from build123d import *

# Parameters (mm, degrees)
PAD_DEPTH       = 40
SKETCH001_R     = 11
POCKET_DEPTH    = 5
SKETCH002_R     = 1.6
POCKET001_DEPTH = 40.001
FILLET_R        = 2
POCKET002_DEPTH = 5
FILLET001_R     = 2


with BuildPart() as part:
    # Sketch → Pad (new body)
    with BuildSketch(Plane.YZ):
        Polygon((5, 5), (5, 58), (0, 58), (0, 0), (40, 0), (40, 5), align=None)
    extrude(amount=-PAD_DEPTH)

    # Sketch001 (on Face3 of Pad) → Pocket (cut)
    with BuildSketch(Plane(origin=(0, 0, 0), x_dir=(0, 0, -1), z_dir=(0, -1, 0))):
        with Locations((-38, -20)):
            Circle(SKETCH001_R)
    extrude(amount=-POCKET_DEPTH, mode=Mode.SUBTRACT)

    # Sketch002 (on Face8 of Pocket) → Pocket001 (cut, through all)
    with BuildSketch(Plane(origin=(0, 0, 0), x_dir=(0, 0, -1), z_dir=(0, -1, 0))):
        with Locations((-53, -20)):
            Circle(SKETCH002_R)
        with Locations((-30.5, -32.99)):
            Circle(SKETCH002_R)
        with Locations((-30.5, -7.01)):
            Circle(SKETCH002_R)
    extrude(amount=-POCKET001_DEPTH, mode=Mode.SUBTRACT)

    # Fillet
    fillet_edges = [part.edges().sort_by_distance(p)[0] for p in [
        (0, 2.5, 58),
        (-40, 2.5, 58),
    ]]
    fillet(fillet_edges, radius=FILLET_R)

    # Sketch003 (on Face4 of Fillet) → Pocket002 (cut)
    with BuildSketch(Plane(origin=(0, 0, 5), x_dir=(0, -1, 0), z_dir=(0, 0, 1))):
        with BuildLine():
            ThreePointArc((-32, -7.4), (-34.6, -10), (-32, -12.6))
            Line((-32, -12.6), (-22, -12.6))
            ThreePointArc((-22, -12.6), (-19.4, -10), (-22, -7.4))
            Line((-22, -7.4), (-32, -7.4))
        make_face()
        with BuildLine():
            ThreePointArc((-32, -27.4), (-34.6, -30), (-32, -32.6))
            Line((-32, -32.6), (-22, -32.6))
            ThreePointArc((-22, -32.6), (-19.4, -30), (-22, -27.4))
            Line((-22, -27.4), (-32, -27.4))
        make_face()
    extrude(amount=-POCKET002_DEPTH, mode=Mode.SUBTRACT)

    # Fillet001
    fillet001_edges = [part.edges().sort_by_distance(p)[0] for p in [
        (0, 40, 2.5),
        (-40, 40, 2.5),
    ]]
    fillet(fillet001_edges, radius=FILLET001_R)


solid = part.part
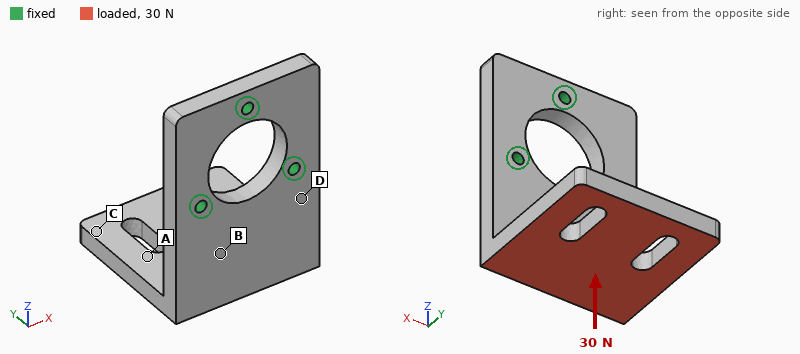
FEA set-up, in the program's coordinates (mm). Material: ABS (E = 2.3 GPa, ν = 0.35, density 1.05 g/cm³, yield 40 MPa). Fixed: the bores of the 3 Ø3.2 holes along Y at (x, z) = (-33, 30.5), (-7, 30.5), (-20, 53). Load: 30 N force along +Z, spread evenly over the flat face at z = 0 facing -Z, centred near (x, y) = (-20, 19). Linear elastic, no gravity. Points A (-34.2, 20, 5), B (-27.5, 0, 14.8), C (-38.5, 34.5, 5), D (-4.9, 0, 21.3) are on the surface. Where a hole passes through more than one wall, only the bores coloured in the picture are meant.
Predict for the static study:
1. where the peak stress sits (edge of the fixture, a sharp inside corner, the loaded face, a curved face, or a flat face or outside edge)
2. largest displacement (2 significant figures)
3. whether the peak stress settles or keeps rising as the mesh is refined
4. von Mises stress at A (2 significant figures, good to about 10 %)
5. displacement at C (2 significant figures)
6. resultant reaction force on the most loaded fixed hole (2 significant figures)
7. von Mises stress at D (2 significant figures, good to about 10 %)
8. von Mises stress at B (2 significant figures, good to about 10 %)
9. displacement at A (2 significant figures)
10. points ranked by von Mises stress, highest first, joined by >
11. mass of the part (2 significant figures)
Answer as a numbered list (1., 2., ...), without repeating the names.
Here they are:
1. edge of the fixture
2. 0.81 mm
3. keeps rising
4. 1.1 MPa
5. 0.66 mm
6. 16 N
7. 3.2 MPa
8. 2.5 MPa
9. 0.38 mm
10. D > B > A > C
11. 17 g
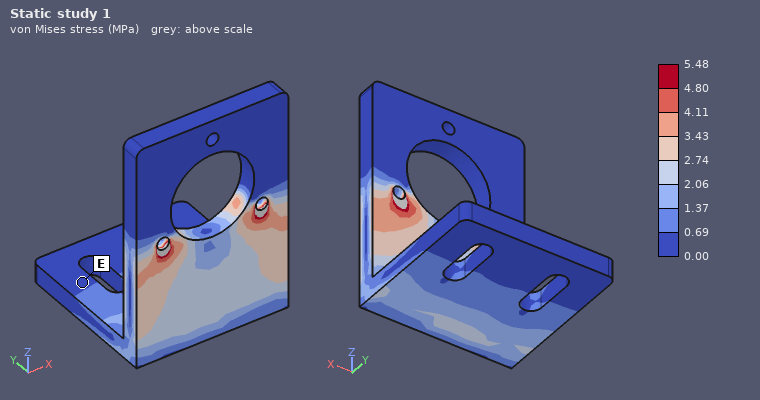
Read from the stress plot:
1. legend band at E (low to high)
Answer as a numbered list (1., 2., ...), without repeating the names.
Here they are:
1. 0.00 to 0.69 MPa
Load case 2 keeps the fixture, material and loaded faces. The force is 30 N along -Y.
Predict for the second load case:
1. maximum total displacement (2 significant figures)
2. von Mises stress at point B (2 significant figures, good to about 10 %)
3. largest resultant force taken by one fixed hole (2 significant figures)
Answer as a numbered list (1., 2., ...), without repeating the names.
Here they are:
1. 0.79 mm
2. 2.3 MPa
3. 16 N
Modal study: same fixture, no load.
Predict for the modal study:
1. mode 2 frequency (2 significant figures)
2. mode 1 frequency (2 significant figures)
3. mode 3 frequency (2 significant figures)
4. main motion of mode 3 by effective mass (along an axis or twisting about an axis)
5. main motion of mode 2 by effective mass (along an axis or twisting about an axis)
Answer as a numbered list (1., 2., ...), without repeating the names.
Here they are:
1. 690 Hz
2. 360 Hz
3. 1000 Hz
4. along Y
5. along X
